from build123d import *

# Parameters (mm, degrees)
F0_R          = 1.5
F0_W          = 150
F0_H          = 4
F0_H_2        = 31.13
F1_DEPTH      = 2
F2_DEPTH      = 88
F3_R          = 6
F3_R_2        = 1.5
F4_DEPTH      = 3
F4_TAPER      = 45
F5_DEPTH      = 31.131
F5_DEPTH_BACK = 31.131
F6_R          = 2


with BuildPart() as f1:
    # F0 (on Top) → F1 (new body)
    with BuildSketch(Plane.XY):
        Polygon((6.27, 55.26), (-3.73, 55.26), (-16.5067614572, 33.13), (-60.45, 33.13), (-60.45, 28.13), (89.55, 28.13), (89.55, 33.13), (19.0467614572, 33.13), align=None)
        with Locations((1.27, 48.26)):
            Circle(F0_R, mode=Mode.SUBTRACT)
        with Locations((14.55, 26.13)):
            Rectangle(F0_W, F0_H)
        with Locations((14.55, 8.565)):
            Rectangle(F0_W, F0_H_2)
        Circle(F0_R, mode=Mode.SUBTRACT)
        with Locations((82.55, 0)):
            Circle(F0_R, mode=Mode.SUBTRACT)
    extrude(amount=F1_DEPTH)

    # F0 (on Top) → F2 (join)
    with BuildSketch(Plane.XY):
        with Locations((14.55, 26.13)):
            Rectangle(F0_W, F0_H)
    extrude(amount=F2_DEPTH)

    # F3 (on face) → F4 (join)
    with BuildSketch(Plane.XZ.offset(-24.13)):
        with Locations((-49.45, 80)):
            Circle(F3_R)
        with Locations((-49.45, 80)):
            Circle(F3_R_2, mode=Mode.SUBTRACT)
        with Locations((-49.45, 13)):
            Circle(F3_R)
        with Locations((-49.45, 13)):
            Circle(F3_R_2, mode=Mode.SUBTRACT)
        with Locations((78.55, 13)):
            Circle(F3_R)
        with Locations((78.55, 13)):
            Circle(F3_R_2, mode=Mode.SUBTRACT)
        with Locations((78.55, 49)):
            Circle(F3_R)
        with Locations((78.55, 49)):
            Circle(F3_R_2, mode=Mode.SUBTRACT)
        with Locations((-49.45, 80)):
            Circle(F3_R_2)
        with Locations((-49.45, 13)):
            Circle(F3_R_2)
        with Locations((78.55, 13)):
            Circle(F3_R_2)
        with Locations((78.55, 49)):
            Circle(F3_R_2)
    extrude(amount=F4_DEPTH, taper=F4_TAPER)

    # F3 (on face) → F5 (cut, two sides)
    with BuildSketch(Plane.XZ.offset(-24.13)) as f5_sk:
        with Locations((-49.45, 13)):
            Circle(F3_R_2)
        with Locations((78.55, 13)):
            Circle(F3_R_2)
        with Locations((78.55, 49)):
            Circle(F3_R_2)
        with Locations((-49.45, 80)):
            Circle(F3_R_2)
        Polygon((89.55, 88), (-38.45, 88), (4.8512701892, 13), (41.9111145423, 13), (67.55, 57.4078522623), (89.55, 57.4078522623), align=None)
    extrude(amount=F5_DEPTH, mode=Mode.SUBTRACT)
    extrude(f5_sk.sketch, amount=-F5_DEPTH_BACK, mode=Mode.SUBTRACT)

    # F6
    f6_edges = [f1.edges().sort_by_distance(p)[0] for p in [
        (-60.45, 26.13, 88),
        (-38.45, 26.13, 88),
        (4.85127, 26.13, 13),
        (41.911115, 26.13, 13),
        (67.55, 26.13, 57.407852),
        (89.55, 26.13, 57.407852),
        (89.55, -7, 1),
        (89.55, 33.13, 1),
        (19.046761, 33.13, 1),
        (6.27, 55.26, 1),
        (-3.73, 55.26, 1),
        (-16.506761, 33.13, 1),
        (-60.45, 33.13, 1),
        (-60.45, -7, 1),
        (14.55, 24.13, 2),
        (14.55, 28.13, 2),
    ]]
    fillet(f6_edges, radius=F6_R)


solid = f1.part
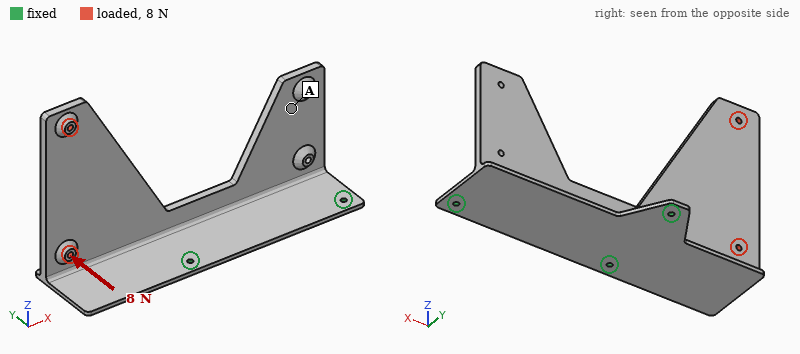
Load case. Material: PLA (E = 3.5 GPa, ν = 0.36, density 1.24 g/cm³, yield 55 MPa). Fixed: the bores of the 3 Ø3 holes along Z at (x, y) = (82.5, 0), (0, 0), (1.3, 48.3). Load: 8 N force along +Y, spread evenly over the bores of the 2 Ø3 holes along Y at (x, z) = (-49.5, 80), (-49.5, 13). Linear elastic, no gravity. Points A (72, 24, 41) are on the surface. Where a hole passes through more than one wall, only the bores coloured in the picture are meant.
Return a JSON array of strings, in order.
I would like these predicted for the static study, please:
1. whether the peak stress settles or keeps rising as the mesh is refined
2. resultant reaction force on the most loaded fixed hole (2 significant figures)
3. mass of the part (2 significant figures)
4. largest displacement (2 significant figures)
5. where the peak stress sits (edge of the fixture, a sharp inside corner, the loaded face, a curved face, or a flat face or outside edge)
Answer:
["keeps rising", "13 N", "49 g", "2.2 mm", "edge of the fixture"]
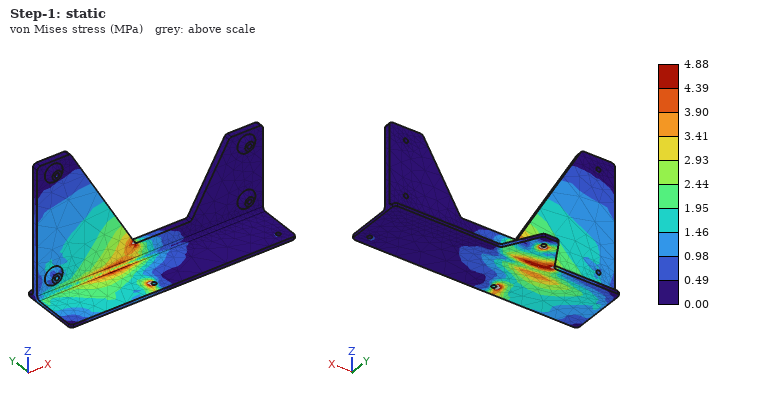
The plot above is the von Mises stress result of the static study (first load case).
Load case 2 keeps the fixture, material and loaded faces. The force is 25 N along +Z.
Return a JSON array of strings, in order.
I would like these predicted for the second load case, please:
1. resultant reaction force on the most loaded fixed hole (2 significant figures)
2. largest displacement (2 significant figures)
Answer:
["34 N", "1.9 mm"]
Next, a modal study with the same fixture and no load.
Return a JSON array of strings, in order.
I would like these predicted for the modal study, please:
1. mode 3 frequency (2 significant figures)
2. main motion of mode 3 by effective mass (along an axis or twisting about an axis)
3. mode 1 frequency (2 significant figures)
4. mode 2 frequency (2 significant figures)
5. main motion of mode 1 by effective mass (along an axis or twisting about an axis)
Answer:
["200 Hz", "along Z", "110 Hz", "120 Hz", "along Y"]
